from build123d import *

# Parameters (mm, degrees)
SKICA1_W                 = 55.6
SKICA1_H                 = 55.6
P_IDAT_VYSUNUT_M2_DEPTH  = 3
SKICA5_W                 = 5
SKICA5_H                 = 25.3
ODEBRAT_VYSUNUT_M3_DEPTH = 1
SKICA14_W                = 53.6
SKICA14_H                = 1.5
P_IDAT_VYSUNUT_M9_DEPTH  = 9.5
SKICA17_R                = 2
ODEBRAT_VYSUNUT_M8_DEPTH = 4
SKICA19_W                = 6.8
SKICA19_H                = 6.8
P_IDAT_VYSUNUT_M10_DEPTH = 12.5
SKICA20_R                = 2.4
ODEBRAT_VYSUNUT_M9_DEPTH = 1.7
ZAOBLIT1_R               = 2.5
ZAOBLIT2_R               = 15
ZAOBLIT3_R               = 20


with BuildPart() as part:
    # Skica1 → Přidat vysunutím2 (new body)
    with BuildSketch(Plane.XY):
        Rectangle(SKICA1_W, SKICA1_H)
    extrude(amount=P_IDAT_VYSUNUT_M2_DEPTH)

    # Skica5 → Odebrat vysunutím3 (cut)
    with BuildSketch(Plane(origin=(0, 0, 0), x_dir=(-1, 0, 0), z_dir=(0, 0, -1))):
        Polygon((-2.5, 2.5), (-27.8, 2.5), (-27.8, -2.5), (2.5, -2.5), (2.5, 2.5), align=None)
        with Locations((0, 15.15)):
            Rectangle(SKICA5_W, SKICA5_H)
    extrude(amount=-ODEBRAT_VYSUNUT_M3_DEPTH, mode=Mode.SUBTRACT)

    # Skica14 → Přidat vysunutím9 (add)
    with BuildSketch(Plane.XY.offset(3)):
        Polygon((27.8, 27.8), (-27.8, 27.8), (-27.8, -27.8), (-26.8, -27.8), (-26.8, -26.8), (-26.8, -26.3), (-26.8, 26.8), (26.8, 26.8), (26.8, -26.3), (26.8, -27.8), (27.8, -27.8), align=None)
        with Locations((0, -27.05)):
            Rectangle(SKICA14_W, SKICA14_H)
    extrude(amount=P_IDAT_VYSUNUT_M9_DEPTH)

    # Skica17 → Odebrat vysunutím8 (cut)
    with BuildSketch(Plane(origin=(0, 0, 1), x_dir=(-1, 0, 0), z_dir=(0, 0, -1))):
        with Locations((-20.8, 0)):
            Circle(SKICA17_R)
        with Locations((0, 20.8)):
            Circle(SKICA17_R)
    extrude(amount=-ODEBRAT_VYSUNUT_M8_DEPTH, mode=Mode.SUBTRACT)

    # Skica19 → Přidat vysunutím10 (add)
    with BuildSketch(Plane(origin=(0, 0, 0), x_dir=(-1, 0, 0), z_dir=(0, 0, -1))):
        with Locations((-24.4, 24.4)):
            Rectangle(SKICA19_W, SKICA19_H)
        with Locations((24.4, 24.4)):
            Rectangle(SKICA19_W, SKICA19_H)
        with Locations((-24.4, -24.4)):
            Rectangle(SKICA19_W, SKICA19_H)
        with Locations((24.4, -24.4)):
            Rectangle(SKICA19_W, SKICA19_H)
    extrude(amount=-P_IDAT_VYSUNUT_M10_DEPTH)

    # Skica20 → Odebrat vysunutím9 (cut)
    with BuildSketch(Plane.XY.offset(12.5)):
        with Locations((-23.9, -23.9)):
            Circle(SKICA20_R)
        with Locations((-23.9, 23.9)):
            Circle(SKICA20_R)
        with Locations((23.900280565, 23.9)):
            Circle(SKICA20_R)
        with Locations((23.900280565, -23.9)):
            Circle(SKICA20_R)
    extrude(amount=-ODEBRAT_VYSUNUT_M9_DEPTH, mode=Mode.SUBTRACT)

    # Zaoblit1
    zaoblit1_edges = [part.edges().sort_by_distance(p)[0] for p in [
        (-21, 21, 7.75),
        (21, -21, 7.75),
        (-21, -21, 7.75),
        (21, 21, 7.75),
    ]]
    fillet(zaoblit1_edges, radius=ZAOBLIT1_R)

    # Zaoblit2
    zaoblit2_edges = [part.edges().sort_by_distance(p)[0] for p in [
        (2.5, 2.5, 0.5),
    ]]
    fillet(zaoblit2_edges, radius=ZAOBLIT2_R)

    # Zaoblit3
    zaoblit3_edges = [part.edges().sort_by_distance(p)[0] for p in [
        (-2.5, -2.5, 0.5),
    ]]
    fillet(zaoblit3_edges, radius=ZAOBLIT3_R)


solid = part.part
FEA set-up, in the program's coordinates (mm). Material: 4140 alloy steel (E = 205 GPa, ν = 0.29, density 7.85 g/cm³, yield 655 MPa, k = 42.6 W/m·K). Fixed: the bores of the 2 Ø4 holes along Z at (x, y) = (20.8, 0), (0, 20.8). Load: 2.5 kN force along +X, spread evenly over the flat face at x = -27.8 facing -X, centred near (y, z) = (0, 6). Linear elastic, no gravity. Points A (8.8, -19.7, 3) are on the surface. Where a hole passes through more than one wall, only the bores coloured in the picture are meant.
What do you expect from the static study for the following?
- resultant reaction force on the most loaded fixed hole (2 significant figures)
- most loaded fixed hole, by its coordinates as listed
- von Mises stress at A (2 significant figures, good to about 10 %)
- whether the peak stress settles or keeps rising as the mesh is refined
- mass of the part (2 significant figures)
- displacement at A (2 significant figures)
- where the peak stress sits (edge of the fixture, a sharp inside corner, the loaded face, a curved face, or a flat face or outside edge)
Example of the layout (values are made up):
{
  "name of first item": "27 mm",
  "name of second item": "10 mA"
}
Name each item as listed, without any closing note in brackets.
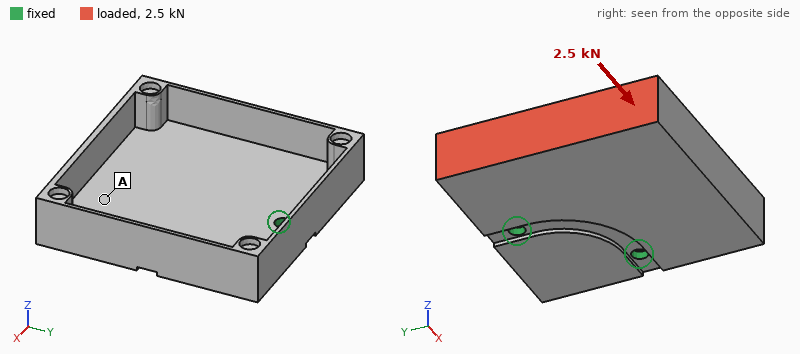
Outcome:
{
  "resultant reaction force on the most loaded fixed hole": "1.8 kN",
  "most loaded fixed hole, by its coordinates as listed": "(20.8, 0)",
  "von Mises stress at A": "55 MPa",
  "whether the peak stress settles or keeps rising as the mesh is refined": "keeps rising",
  "mass of the part": "97 g",
  "displacement at A": "0.060 mm",
  "where the peak stress sits": "edge of the fixture"
}
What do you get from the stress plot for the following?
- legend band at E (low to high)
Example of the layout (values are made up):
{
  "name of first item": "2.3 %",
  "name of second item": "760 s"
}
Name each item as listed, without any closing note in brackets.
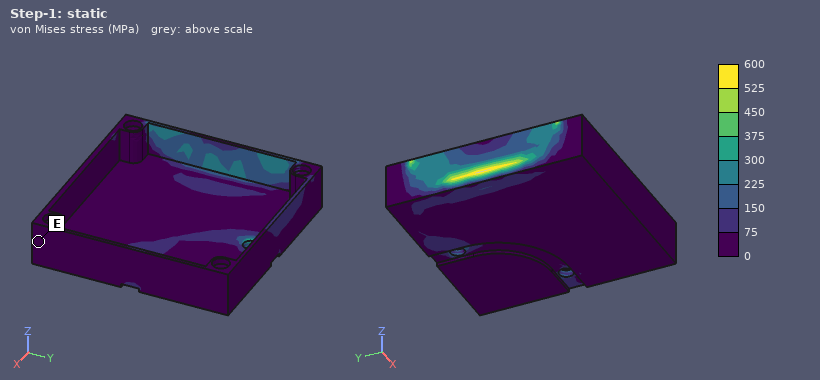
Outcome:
{
  "legend band at E": "0 to 75 MPa"
}
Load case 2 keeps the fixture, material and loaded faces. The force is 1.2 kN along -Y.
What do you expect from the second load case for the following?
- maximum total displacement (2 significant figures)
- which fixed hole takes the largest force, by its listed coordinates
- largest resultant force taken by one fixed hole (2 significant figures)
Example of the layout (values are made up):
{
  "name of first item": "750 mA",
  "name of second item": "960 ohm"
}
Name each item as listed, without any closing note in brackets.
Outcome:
{
  "maximum total displacement": "0.21 mm",
  "which fixed hole takes the largest force, by its listed coordinates": "(0, 20.8)",
  "largest resultant force taken by one fixed hole": "1.9 kN"
}
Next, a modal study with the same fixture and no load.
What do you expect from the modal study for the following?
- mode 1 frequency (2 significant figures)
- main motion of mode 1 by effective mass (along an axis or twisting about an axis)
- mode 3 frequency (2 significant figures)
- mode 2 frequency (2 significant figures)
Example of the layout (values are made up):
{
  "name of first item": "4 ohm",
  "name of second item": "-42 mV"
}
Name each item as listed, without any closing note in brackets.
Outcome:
{
  "mode 1 frequency": "960 Hz",
  "main motion of mode 1 by effective mass": "along Z",
  "mode 3 frequency": "3400 Hz",
  "mode 2 frequency": "3000 Hz"
}
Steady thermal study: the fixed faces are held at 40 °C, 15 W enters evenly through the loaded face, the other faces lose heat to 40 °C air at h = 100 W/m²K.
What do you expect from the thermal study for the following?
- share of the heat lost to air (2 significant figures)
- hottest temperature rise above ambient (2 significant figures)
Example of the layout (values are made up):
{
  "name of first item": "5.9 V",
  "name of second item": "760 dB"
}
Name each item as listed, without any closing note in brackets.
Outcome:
{
  "share of the heat lost to air": "78 %",
  "hottest temperature rise above ambient": "51 K"
}
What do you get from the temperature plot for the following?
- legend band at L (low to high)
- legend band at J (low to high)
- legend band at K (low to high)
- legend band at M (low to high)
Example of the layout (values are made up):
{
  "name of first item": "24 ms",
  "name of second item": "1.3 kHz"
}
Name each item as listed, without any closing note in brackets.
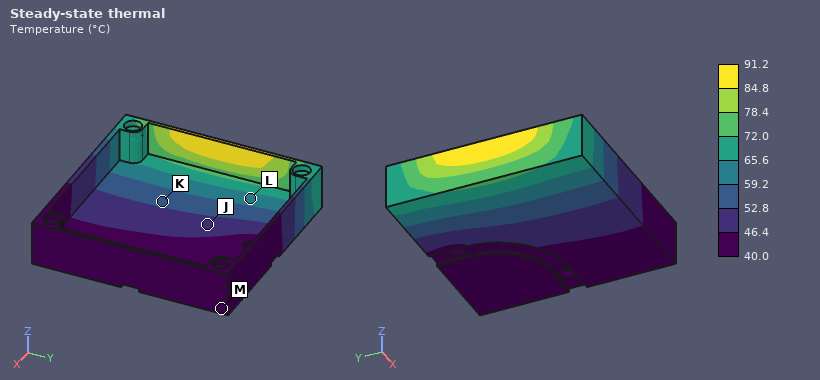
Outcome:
{
  "legend band at L": "59.2 to 65.6 °C",
  "legend band at J": "46.4 to 52.8 °C",
  "legend band at K": "52.8 to 59.2 °C",
  "legend band at M": "40.0 to 46.4 °C"
}
